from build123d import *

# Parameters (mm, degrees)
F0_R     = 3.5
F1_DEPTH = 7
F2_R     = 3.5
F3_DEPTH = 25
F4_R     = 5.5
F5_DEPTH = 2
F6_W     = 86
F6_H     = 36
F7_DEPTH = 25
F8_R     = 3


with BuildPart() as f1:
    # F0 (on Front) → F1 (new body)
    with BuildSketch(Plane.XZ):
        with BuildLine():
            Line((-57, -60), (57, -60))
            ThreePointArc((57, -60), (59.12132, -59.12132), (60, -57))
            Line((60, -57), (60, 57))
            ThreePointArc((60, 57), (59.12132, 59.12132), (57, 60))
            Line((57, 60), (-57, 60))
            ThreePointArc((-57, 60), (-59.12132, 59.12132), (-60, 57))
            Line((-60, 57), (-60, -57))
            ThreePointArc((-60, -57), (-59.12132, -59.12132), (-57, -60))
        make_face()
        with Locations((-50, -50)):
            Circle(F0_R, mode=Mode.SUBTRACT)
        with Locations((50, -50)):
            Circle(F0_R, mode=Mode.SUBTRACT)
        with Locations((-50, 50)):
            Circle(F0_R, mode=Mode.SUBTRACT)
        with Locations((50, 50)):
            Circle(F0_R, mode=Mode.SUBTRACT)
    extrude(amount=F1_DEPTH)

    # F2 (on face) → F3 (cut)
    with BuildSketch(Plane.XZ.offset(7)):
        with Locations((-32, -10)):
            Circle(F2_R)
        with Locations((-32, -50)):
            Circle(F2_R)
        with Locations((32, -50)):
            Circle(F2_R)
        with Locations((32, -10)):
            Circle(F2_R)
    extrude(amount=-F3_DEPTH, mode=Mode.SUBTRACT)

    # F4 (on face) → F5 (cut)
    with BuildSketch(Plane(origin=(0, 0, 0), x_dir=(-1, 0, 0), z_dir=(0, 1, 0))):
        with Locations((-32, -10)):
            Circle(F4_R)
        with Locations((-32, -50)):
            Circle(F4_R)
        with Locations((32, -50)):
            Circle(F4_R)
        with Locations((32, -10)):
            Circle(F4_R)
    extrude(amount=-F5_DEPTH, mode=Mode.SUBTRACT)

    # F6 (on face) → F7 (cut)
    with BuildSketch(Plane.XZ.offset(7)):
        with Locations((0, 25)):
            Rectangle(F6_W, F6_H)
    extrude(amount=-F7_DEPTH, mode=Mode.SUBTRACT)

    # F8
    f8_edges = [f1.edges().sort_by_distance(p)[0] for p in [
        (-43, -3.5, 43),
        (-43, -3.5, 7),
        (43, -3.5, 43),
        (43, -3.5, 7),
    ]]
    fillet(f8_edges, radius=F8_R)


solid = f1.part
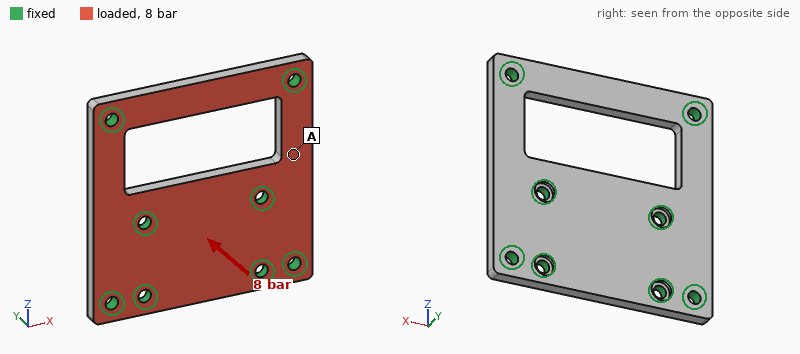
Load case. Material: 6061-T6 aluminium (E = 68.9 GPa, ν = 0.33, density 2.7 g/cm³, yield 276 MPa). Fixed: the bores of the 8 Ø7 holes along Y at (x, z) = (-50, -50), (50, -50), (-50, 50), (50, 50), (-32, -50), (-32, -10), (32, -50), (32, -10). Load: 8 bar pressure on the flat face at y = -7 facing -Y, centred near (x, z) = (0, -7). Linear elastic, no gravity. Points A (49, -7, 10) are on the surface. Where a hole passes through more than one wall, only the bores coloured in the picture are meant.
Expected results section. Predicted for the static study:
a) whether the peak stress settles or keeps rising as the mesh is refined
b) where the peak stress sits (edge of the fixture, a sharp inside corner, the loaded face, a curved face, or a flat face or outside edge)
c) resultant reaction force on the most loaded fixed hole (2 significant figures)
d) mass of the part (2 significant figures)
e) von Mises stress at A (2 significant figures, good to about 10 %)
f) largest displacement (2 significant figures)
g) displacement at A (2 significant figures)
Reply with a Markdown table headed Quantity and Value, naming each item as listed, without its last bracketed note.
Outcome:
| Quantity | Value |
|---|---|
| whether the peak stress settles or keeps rising as the mesh is refined | keeps rising |
| where the peak stress sits | edge of the fixture |
| resultant reaction force on the most loaded fixed hole | 1.8 kN |
| mass of the part | 210 g |
| von Mises stress at A | 13 MPa |
| largest displacement | 92 µm |
| displacement at A | 21 µm |
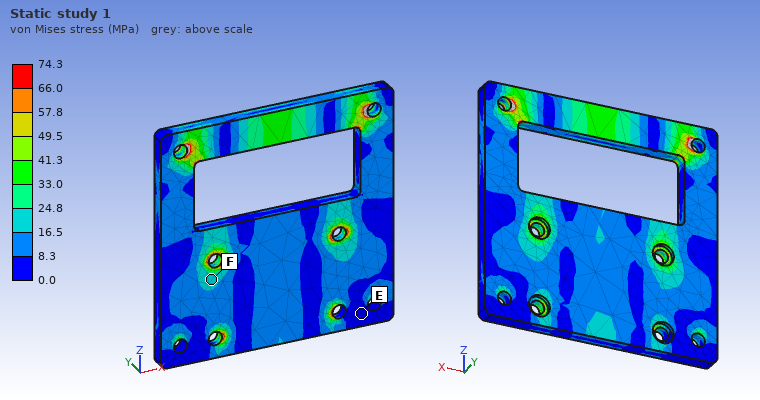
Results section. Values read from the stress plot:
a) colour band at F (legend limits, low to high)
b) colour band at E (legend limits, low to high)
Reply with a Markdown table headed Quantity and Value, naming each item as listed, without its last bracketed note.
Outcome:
| Quantity | Value |
|---|---|
| colour band at F | 16.5 to 24.8 MPa |
| colour band at E | 0.0 to 8.3 MPa |
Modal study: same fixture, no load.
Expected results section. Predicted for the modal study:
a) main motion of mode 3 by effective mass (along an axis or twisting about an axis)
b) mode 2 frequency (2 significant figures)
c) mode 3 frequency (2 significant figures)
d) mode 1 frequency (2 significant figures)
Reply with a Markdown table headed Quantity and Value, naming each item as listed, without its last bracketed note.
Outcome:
| Quantity | Value |
|---|---|
| main motion of mode 3 by effective mass | twisting about Z |
| mode 2 frequency | 6600 Hz |
| mode 3 frequency | 6900 Hz |
| mode 1 frequency | 3900 Hz |
